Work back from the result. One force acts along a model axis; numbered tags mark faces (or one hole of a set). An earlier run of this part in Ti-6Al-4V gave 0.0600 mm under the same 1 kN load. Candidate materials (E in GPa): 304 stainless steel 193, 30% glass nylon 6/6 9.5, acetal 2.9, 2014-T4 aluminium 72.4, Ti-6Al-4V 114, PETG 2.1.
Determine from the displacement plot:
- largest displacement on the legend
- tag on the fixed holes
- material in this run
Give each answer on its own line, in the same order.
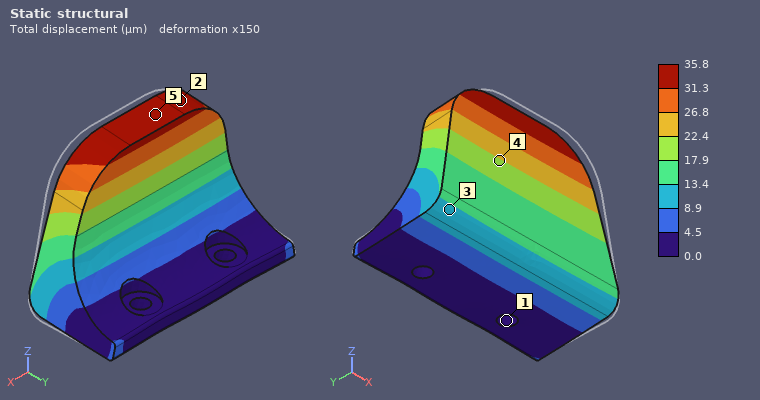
35.8 µm
1
304 stainless steel
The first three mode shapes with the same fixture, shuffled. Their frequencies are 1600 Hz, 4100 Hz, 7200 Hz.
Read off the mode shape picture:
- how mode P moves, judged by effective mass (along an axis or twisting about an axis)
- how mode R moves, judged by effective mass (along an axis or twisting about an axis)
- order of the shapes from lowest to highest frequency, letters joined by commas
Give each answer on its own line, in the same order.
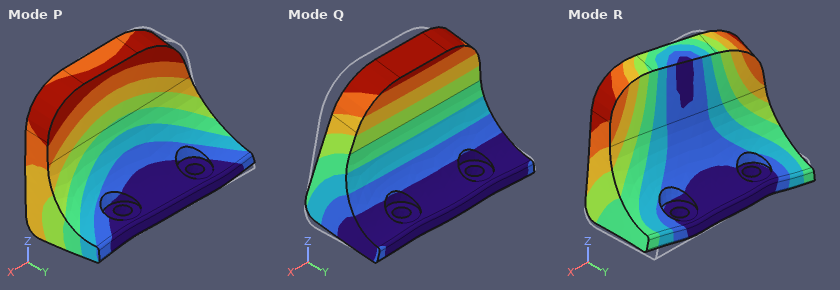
along X
along X
Q, P, R
